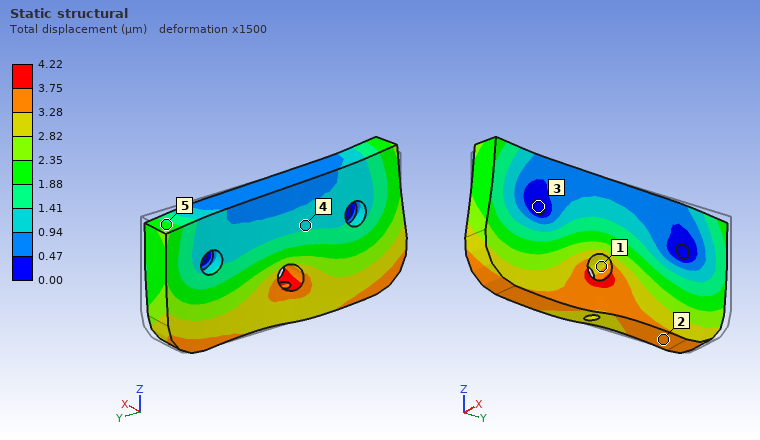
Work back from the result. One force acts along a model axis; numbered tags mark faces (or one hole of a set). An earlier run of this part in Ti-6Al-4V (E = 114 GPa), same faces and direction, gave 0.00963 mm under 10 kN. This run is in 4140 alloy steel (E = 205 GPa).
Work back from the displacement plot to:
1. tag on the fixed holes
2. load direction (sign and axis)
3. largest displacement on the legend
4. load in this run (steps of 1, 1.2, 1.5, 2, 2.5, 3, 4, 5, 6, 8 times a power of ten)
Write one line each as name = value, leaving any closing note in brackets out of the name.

tag on the fixed holes = 3
load direction = -Y
largest displacement on the legend = 4.22 µm
load in this run = 8 kN
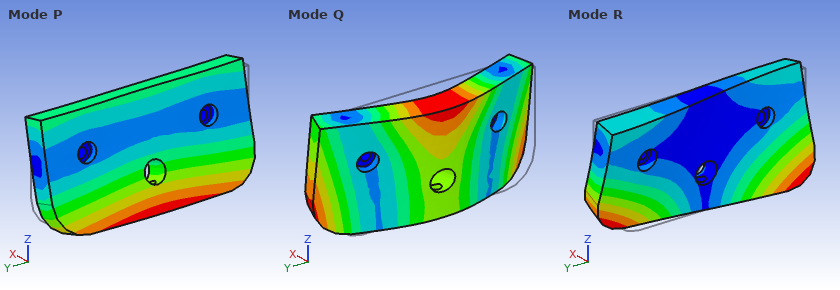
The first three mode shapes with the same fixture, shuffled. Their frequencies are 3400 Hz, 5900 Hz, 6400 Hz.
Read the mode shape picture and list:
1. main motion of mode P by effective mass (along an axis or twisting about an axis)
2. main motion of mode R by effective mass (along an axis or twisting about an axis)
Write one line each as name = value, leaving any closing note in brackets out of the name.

main motion of mode P by effective mass = along X
main motion of mode R by effective mass = twisting about Z
